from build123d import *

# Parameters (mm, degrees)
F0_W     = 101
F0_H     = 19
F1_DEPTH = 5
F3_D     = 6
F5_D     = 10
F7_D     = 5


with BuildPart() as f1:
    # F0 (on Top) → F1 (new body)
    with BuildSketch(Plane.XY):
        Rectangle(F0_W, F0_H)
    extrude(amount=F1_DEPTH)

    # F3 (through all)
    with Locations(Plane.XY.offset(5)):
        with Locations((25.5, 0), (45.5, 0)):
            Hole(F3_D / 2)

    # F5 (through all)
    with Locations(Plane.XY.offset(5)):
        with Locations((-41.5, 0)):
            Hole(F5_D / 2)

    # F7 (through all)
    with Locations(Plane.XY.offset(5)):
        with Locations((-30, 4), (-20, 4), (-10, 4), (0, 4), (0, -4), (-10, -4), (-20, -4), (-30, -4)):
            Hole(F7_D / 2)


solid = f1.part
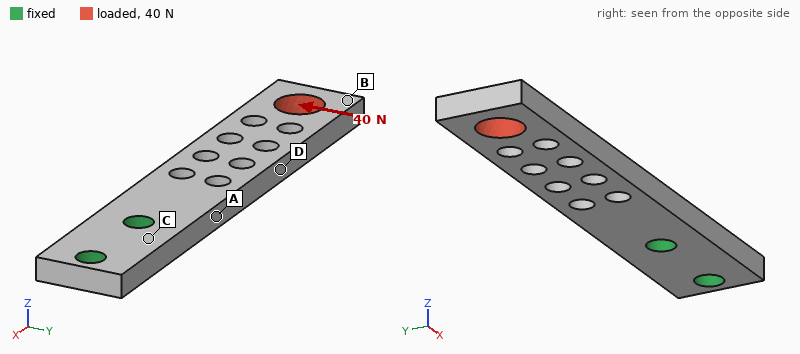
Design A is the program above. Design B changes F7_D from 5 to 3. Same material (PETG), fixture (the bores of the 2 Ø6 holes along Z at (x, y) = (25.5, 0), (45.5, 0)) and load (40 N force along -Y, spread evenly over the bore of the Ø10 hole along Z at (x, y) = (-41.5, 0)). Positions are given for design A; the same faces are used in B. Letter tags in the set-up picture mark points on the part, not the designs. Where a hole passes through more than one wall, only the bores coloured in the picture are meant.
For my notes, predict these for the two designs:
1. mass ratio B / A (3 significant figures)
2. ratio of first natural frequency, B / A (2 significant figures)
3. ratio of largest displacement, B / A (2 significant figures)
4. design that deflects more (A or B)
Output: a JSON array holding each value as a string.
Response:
["1.06", "1.0", "0.92", "A"]
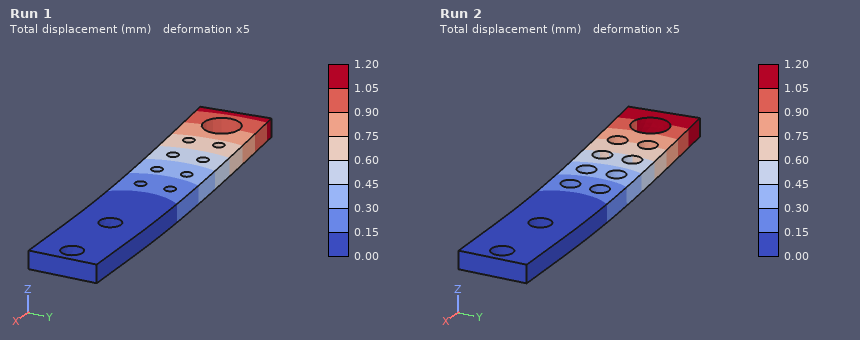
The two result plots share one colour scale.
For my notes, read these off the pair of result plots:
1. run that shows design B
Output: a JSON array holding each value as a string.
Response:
["Run 1"]
